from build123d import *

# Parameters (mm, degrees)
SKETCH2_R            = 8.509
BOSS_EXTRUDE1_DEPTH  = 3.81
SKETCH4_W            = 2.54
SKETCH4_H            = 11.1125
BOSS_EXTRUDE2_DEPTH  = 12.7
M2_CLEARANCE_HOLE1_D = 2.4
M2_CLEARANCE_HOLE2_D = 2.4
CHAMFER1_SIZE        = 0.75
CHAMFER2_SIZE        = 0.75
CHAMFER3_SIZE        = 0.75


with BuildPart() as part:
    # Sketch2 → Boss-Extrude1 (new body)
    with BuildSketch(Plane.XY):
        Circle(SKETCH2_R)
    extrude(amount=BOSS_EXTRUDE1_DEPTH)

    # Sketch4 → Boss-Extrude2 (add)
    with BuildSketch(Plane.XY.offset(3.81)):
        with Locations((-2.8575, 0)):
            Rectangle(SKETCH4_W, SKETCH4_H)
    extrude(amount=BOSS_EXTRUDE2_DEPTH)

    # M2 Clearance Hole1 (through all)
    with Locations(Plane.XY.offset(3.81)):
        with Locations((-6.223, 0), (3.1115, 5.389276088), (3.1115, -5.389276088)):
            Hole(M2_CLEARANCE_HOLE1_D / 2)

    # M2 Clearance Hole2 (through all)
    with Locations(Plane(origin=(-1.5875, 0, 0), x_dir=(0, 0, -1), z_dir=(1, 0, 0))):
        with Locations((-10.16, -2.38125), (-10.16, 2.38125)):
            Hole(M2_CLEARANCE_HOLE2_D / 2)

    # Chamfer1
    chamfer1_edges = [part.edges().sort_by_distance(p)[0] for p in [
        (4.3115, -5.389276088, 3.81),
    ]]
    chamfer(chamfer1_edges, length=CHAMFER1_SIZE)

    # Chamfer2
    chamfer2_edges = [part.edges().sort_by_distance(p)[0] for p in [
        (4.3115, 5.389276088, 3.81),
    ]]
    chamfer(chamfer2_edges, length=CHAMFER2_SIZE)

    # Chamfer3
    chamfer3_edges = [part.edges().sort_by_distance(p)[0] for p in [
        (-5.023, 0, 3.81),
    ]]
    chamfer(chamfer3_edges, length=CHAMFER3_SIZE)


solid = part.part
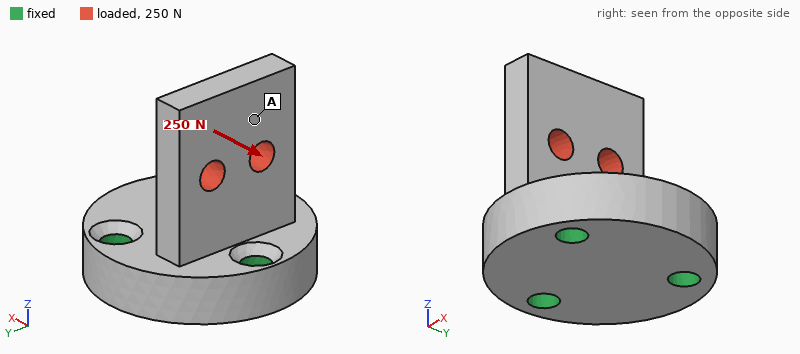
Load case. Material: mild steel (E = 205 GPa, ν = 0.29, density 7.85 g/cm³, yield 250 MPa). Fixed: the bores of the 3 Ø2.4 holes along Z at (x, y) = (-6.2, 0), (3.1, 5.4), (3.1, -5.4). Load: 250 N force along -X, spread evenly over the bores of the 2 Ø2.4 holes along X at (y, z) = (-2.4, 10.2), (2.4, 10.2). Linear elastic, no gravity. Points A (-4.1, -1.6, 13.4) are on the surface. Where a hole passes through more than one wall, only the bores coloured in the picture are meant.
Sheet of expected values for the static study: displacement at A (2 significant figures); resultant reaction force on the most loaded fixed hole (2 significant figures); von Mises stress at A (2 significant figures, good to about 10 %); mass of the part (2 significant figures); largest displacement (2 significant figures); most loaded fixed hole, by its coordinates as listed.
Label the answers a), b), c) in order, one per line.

a) 18 µm
b) 270 N
c) 10.0 MPa
d) 9.0 g
e) 25 µm
f) (-6.2, 0)
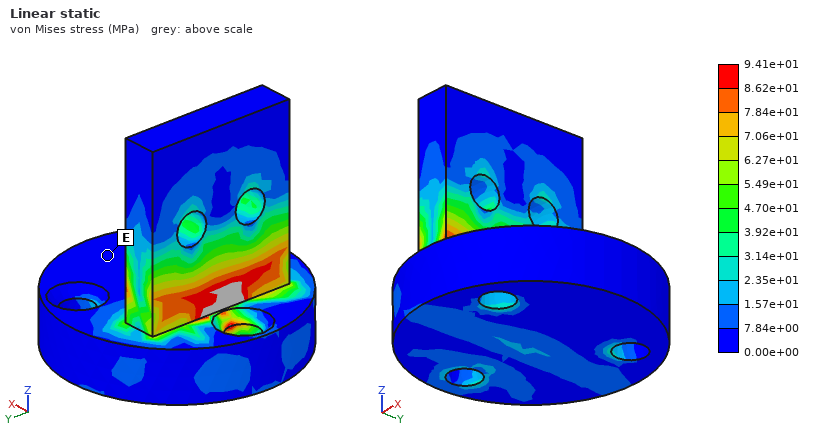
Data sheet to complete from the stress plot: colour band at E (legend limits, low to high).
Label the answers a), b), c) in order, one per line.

a) 0.00e+00 to 7.84e+00 MPa
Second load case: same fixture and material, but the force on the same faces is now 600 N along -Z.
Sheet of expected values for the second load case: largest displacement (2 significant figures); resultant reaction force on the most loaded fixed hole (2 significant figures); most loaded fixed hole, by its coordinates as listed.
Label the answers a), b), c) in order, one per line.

a) 1.6 µm
b) 370 N
c) (-6.2, 0)
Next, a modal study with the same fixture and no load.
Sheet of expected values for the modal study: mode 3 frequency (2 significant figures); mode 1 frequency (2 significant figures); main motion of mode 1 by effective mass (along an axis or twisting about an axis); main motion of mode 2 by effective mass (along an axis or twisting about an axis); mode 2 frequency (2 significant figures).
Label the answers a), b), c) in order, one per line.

a) 28 kHz
b) 11 kHz
c) along X
d) along Y
e) 25 kHz
